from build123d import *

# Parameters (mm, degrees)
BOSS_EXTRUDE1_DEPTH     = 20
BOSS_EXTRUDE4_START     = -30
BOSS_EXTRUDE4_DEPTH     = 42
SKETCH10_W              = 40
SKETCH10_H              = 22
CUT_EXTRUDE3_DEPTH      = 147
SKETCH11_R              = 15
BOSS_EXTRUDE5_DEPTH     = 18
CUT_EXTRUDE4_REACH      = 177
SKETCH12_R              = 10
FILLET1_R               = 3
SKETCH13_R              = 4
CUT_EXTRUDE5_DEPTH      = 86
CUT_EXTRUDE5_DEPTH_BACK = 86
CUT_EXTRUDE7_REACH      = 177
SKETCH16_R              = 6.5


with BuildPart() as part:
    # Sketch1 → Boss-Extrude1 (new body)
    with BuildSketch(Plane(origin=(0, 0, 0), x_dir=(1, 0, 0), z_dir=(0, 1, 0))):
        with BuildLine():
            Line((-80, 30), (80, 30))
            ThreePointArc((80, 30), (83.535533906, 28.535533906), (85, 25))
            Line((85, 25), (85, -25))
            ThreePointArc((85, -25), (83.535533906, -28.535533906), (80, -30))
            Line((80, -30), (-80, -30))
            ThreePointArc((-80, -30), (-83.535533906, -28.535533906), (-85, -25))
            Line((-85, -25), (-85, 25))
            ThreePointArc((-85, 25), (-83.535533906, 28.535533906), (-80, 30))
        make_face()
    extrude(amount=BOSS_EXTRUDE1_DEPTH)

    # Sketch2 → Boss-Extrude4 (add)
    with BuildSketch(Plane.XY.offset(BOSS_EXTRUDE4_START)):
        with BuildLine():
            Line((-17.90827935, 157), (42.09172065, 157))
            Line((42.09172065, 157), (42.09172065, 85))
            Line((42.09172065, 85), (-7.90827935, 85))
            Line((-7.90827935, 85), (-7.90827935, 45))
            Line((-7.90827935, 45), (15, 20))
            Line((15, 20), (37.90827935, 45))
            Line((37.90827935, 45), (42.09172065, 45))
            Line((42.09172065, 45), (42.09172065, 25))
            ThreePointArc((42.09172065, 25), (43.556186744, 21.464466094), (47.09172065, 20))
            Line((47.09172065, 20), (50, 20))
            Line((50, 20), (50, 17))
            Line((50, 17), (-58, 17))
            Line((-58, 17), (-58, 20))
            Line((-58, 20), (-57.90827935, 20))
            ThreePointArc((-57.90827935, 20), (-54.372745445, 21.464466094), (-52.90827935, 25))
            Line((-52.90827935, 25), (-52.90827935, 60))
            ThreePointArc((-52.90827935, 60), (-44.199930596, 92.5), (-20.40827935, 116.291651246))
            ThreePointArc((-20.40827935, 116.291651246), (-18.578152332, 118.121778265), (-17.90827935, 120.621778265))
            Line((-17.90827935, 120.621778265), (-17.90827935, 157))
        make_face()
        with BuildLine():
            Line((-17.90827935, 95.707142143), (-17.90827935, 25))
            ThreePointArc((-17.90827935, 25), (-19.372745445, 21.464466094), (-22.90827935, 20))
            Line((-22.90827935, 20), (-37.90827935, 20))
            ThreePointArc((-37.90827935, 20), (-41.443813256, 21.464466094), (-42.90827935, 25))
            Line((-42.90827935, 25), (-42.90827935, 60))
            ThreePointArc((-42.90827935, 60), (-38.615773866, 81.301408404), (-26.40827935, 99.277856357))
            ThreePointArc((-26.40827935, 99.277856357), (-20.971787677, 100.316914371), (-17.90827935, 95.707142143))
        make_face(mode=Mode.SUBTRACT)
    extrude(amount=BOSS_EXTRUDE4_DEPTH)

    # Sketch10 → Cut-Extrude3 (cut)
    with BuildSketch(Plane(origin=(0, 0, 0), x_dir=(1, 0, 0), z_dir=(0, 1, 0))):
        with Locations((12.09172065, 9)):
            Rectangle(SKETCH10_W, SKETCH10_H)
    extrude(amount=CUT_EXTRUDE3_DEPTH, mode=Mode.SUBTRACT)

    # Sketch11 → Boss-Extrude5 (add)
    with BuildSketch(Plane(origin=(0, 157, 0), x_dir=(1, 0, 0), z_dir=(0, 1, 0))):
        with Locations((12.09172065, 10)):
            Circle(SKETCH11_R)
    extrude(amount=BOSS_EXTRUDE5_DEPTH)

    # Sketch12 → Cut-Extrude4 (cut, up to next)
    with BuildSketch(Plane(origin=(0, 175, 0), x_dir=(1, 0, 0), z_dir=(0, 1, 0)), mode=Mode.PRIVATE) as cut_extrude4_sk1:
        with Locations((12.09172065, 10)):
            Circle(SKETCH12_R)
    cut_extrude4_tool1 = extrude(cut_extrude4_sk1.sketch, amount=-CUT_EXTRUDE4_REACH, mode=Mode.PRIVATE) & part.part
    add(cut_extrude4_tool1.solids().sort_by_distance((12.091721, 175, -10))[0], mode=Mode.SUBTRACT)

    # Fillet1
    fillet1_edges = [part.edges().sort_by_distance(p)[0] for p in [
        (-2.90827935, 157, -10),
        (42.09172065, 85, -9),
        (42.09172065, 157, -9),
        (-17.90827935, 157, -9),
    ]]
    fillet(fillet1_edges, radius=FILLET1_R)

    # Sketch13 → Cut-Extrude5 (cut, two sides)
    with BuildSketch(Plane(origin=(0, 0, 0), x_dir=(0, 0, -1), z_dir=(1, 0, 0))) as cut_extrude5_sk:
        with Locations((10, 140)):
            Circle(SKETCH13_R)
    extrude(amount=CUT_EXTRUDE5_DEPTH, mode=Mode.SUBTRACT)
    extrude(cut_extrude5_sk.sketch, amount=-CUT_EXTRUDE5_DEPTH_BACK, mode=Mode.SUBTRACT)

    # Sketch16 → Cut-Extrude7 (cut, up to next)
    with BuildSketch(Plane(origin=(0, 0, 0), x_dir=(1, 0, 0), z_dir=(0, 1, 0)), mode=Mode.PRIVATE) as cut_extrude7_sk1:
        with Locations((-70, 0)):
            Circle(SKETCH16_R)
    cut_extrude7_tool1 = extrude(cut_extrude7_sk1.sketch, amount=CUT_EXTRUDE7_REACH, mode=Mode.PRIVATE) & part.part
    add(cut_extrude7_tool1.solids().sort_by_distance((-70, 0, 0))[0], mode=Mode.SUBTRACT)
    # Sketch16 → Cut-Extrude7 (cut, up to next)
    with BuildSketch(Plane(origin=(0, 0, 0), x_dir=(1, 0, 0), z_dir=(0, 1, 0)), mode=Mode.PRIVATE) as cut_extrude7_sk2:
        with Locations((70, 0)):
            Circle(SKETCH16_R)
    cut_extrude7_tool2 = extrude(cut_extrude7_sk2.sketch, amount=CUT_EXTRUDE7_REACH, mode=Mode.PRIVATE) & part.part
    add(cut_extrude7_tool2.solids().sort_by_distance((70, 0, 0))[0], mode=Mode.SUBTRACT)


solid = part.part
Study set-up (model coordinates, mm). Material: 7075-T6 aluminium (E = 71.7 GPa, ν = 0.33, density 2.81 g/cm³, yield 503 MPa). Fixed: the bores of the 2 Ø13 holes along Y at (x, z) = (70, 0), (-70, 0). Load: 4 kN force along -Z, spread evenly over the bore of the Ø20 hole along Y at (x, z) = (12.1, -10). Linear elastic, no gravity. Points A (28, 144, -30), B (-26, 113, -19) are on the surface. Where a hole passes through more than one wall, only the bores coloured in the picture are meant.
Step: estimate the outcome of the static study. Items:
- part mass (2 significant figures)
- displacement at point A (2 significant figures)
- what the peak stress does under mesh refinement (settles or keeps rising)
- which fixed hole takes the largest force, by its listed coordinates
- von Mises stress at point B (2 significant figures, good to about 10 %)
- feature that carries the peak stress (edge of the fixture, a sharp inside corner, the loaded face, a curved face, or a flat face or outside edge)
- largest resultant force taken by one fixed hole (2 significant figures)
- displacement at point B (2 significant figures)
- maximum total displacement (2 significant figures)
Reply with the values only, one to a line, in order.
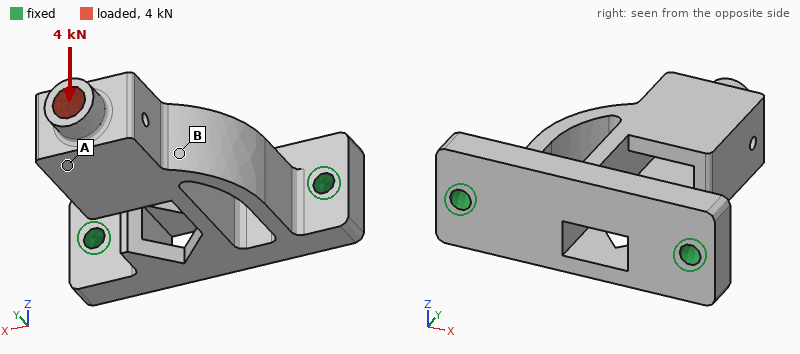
1.1 kg
1.3 mm
keeps rising
(70, 0)
54 MPa
edge of the fixture
2.3 kN
0.65 mm
1.6 mm
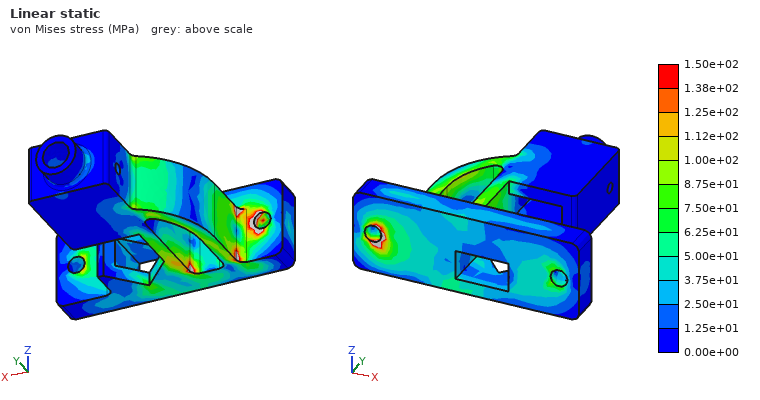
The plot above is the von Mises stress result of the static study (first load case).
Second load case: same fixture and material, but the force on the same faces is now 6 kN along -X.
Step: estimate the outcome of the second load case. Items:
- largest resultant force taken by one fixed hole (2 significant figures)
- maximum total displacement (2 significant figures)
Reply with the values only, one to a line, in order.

7.9 kN
1.3 mm
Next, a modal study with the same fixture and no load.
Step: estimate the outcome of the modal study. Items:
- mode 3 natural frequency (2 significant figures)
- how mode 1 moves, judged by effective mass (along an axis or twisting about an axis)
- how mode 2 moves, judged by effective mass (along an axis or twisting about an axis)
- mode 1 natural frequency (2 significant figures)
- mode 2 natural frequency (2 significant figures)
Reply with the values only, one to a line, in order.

1700 Hz
along Z
along X
550 Hz
740 Hz
